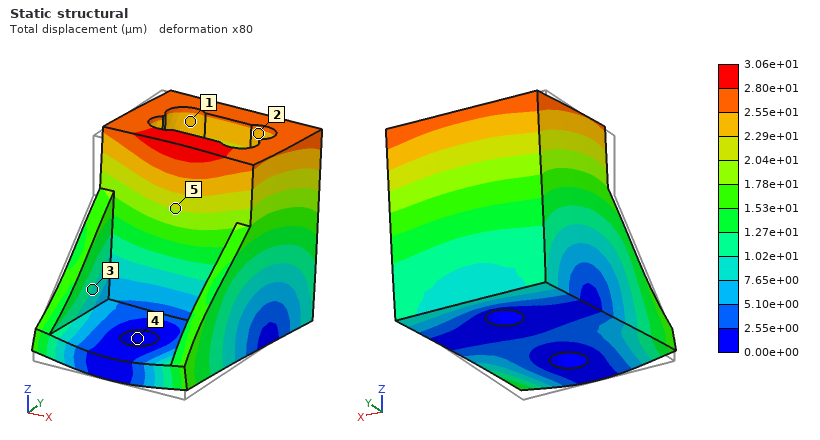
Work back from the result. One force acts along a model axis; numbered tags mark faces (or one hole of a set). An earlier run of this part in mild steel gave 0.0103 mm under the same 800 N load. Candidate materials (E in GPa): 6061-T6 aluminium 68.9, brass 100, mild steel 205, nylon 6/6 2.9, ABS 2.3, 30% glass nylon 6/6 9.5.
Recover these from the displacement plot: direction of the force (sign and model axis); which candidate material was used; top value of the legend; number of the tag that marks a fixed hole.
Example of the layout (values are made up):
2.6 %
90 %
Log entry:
+Y
6061-T6 aluminium
3.06e+01 µm
4
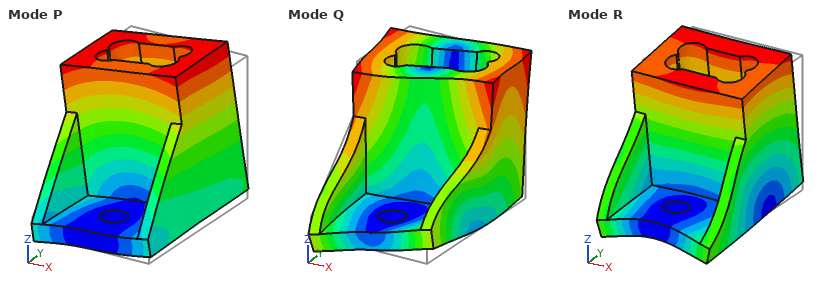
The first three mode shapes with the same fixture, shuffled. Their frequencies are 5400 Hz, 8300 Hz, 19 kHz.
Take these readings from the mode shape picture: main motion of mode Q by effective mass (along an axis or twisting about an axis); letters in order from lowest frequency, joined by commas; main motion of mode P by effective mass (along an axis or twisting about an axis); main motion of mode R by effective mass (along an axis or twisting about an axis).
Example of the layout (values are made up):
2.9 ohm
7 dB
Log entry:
twisting about Z
P, R, Q
along X
along Y
